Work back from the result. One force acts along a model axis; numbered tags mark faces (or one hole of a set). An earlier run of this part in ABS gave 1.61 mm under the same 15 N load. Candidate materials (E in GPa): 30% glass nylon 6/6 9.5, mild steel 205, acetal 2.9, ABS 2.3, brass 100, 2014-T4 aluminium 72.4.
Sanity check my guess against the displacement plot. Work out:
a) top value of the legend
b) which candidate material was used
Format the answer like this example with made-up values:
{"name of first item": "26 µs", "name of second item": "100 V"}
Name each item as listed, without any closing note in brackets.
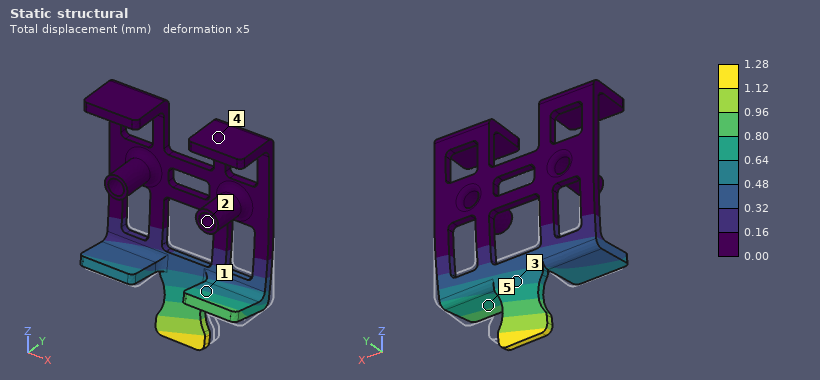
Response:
{"top value of the legend": "1.28 mm", "which candidate material was used": "acetal"}
